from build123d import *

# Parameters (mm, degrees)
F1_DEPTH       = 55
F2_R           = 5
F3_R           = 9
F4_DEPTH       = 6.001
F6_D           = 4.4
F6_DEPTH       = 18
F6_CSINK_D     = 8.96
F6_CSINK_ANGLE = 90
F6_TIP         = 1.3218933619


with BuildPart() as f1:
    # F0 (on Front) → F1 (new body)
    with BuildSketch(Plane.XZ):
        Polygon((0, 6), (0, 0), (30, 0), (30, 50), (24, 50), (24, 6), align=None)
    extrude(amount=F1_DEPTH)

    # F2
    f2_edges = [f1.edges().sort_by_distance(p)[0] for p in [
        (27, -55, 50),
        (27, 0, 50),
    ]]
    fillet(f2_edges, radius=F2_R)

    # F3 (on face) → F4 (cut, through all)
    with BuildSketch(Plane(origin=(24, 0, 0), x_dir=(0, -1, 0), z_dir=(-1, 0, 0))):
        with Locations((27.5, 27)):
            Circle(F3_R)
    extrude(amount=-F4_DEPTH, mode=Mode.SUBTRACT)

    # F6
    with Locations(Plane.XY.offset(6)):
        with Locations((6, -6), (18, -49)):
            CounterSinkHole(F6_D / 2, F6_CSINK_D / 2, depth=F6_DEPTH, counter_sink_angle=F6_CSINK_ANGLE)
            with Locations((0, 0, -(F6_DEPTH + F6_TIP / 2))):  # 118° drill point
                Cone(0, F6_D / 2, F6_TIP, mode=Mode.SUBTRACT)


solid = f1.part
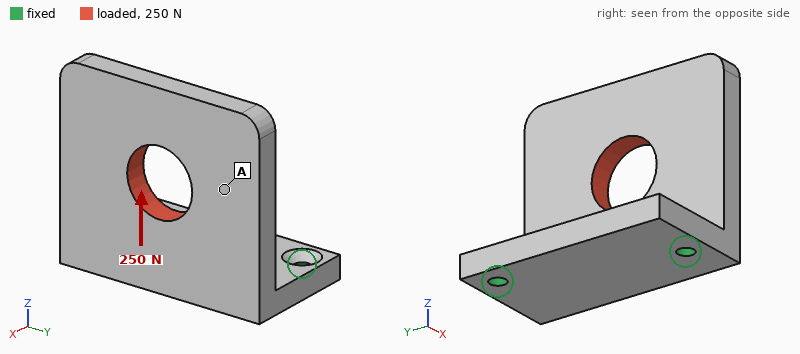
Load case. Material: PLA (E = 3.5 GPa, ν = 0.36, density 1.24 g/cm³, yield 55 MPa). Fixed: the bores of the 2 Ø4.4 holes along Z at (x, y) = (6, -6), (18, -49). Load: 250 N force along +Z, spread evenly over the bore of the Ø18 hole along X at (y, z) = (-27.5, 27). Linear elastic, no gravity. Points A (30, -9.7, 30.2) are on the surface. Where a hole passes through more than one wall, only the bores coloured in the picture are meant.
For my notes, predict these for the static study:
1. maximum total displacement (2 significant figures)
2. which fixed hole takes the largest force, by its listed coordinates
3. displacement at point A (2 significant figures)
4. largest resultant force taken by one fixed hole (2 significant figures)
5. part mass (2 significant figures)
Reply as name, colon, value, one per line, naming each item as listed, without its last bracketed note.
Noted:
maximum total displacement: 0.91 mm
which fixed hole takes the largest force, by its listed coordinates: (18, -49)
displacement at point A: 0.61 mm
largest resultant force taken by one fixed hole: 150 N
part mass: 28 g
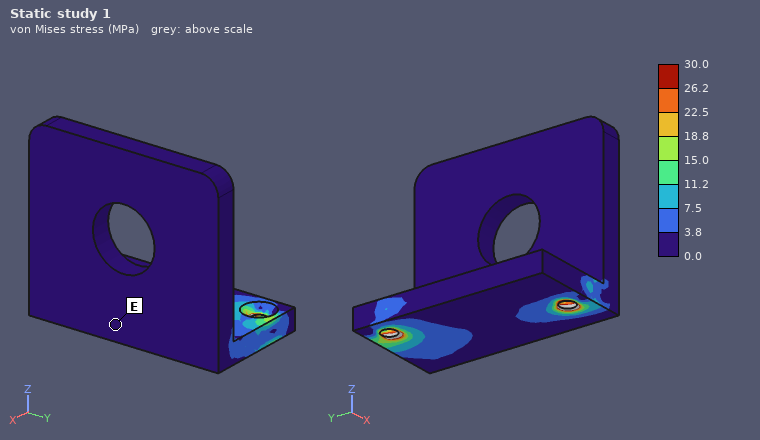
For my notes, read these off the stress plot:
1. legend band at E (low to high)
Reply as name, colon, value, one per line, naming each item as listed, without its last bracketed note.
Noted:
legend band at E: 0.0 to 3.8 MPa
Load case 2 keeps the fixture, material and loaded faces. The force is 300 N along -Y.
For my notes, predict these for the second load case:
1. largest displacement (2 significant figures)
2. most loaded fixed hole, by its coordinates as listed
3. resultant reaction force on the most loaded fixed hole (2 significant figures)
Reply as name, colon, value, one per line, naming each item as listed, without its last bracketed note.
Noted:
largest displacement: 0.81 mm
most loaded fixed hole, by its coordinates as listed: (18, -49)
resultant reaction force on the most loaded fixed hole: 250 N
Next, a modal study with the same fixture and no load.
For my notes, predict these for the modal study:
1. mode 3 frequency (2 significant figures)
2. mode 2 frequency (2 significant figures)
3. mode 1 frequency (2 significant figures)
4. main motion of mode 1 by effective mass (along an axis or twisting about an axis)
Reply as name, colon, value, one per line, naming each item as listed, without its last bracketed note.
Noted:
mode 3 frequency: 1400 Hz
mode 2 frequency: 1000 Hz
mode 1 frequency: 440 Hz
main motion of mode 1 by effective mass: along X
